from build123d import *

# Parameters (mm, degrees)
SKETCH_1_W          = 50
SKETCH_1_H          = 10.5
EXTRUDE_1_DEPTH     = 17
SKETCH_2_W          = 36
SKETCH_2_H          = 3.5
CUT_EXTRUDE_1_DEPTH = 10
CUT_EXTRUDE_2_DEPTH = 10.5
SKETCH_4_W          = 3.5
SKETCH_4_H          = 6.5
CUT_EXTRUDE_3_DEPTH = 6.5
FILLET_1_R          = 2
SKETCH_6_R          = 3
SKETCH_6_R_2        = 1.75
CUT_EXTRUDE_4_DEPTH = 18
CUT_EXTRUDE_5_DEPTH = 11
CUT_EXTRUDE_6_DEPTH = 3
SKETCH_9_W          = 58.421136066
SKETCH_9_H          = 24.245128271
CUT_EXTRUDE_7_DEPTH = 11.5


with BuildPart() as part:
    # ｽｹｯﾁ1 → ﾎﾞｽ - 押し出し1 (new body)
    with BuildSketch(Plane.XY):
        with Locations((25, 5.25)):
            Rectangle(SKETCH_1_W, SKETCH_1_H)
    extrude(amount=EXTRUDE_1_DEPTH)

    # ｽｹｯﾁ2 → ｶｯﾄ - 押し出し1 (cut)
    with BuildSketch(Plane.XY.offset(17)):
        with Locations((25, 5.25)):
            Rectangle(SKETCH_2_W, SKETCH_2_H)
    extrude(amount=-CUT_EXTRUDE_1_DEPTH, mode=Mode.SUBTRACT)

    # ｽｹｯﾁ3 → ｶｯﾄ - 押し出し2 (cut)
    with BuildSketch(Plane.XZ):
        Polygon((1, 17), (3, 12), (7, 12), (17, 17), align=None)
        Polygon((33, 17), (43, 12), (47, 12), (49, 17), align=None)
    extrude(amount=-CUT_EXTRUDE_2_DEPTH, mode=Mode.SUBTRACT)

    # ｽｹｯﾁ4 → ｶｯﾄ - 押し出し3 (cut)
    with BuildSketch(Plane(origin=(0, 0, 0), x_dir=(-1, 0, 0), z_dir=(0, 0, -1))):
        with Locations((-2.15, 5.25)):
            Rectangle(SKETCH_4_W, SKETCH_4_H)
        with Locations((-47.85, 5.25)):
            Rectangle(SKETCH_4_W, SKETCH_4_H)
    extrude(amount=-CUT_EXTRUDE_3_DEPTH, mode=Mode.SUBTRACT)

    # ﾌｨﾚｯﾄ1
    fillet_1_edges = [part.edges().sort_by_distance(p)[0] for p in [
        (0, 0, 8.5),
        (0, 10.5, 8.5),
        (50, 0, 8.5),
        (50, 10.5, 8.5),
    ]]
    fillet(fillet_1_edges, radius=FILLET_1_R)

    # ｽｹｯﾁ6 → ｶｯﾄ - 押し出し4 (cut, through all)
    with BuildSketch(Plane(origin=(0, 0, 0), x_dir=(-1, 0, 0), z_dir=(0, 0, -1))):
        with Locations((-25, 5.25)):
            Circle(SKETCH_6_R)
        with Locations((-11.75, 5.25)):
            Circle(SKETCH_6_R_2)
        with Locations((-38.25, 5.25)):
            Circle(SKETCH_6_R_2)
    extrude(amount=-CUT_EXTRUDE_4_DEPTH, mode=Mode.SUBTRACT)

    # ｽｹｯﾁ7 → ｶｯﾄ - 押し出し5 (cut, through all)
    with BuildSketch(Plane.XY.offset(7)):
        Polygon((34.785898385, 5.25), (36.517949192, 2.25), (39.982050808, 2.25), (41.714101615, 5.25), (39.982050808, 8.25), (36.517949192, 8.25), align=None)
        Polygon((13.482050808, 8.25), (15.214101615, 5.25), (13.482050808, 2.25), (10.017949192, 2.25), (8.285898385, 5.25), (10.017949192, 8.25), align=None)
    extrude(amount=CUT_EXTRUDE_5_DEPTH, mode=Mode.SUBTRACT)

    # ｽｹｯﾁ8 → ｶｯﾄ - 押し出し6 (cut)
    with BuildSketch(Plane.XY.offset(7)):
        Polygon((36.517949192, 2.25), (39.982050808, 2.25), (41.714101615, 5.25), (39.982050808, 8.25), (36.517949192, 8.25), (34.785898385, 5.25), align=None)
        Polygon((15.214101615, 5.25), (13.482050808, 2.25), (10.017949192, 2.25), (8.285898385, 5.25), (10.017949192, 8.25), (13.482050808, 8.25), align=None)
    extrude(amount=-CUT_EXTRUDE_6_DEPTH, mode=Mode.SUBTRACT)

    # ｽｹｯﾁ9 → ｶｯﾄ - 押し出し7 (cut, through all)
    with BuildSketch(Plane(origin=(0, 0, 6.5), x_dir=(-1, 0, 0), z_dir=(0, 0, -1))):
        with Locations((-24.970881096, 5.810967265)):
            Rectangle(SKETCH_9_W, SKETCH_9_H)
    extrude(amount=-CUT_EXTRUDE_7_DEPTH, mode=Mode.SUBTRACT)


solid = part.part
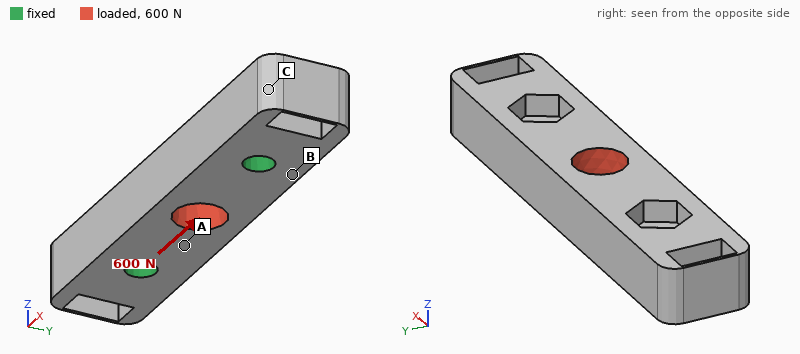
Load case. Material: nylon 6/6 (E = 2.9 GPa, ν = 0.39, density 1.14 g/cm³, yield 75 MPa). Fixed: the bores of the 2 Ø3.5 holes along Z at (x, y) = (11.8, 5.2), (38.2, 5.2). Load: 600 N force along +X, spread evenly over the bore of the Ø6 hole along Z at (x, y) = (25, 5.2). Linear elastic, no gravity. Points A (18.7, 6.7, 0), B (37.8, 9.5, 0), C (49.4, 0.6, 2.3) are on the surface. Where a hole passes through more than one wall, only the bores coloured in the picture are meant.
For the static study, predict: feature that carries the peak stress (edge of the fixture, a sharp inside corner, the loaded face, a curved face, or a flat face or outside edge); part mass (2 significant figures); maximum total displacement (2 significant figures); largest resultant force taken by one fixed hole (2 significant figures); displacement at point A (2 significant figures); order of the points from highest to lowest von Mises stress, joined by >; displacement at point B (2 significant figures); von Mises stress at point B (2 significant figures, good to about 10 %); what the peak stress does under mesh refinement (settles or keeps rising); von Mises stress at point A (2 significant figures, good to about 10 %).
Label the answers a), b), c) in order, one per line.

a) edge of the fixture
b) 3.1 g
c) 27 µm
d) 300 N
e) 14 µm
f) A > B > C
g) 5.9 µm
h) 2.9 MPa
i) keeps rising
j) 7.0 MPa
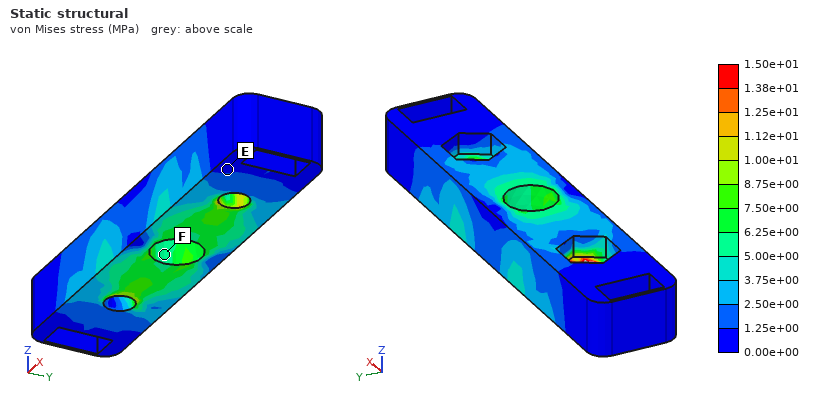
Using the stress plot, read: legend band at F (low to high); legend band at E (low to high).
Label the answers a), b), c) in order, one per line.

a) 5.00e+00 to 6.25e+00 MPa
b) 0.00e+00 to 1.25e+00 MPa
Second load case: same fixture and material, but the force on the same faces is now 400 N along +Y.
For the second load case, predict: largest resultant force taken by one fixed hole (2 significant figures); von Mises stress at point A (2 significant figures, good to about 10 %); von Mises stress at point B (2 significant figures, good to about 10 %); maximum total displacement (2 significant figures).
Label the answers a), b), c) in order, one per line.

a) 200 N
b) 7.0 MPa
c) 4.3 MPa
d) 97 µm
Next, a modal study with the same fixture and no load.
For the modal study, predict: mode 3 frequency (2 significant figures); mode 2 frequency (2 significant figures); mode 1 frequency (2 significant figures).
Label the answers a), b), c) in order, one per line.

a) 10 kHz
b) 9900 Hz
c) 8800 Hz
